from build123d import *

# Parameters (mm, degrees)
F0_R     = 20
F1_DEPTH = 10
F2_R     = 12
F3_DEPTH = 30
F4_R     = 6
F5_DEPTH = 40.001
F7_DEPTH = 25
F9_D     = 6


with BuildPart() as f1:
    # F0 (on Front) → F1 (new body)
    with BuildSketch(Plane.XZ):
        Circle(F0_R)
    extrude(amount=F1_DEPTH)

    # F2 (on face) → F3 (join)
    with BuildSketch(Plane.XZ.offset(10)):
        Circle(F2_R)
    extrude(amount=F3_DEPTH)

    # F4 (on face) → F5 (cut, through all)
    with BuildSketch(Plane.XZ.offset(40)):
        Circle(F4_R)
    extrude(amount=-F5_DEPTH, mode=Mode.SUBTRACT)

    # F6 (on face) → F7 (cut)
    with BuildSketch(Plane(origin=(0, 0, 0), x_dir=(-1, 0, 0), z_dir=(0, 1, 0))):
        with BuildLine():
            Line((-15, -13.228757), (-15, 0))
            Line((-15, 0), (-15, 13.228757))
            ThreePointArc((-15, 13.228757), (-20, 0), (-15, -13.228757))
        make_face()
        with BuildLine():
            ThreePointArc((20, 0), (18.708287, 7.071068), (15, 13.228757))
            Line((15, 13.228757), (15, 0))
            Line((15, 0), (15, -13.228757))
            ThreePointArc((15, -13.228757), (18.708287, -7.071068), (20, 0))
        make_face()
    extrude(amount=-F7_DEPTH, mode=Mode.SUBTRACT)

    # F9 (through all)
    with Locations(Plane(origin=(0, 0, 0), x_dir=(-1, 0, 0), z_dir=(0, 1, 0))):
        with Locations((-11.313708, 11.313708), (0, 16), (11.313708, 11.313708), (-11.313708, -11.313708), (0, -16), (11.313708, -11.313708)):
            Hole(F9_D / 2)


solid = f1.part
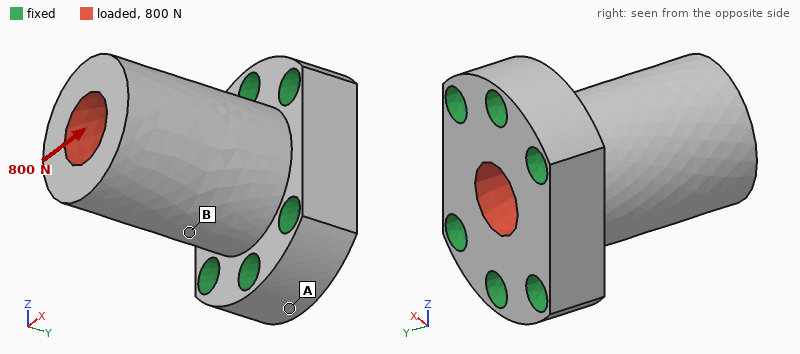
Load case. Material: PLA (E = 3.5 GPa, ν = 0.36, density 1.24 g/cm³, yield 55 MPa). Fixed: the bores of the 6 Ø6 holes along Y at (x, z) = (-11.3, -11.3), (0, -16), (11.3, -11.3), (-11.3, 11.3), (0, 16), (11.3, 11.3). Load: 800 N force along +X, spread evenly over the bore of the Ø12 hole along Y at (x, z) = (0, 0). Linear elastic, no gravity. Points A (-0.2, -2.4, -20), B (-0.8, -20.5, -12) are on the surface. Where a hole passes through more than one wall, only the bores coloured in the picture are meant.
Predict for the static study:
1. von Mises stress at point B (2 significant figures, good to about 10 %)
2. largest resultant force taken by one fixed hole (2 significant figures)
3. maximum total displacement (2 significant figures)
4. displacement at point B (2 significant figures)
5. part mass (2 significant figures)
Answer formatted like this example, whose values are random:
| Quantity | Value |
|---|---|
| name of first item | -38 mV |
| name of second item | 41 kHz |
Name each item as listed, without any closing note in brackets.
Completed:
| Quantity | Value |
|---|---|
| von Mises stress at point B | 2.7 MPa |
| largest resultant force taken by one fixed hole | 330 N |
| maximum total displacement | 0.11 mm |
| displacement at point B | 0.040 mm |
| part mass | 22 g |
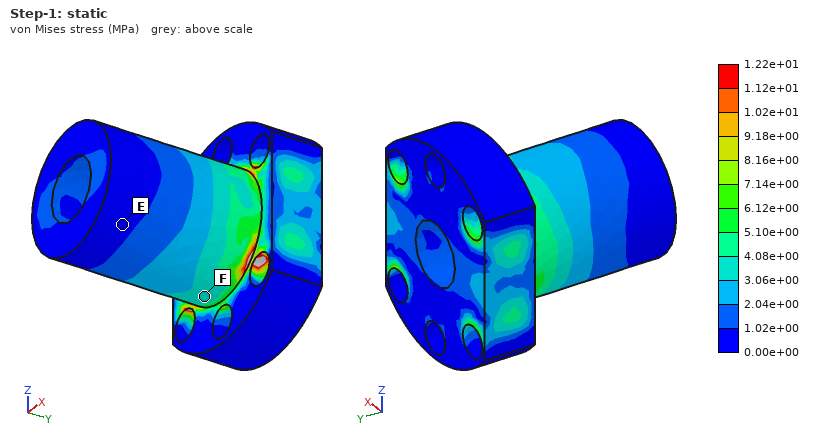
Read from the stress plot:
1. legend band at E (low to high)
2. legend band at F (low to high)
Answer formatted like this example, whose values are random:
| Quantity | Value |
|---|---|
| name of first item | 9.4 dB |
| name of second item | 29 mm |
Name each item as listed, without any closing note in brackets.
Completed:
| Quantity | Value |
|---|---|
| legend band at E | 0.00e+00 to 1.02e+00 MPa |
| legend band at F | 3.06e+00 to 4.08e+00 MPa |
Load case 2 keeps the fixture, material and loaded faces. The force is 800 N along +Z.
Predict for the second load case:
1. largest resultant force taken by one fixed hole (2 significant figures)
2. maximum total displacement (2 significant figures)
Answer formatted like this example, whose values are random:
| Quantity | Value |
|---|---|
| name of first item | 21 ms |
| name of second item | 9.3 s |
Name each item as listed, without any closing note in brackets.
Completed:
| Quantity | Value |
|---|---|
| largest resultant force taken by one fixed hole | 280 N |
| maximum total displacement | 95 µm |
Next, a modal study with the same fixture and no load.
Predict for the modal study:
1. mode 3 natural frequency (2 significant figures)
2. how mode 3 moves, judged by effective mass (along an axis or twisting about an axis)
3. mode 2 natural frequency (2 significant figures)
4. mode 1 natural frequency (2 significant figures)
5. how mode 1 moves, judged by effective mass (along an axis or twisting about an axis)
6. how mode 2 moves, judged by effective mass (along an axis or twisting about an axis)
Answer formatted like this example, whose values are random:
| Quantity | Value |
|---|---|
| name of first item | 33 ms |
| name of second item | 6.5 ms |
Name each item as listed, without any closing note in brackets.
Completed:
| Quantity | Value |
|---|---|
| mode 3 natural frequency | 7800 Hz |
| how mode 3 moves, judged by effective mass | twisting about Y |
| mode 2 natural frequency | 4200 Hz |
| mode 1 natural frequency | 3900 Hz |
| how mode 1 moves, judged by effective mass | along X |
| how mode 2 moves, judged by effective mass | along Z |
